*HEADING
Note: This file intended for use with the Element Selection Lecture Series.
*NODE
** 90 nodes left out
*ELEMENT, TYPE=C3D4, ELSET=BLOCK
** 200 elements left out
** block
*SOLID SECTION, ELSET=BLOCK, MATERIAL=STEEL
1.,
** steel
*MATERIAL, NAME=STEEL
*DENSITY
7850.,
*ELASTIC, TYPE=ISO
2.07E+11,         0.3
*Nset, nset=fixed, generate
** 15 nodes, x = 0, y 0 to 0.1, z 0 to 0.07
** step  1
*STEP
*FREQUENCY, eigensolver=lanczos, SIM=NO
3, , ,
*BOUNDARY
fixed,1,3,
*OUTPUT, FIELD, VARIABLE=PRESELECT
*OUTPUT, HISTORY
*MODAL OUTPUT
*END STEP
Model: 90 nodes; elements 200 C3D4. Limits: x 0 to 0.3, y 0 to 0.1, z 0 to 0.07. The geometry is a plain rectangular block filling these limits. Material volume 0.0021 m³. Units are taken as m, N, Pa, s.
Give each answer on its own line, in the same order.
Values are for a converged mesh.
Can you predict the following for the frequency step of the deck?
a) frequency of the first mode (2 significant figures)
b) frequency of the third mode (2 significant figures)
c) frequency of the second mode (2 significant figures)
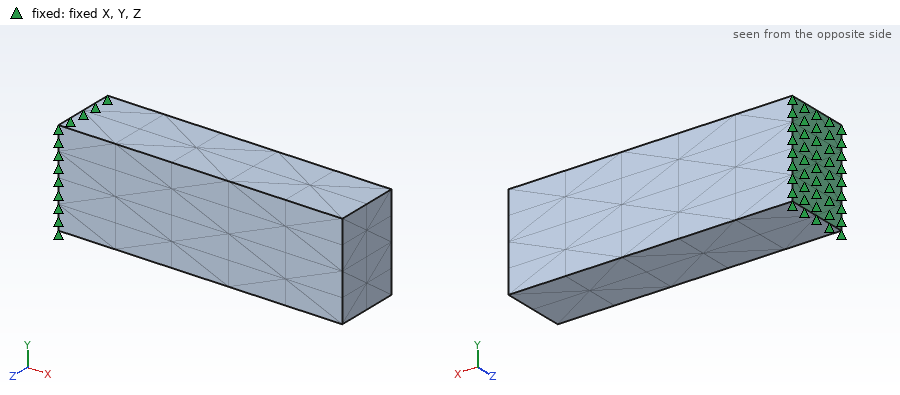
630 Hz
2300 Hz
860 Hz
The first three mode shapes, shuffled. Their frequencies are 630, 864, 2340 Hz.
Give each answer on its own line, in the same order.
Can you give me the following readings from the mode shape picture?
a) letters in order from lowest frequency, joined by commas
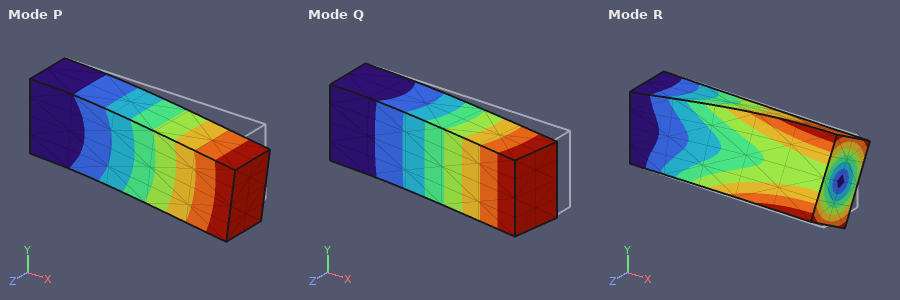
Q, P, R
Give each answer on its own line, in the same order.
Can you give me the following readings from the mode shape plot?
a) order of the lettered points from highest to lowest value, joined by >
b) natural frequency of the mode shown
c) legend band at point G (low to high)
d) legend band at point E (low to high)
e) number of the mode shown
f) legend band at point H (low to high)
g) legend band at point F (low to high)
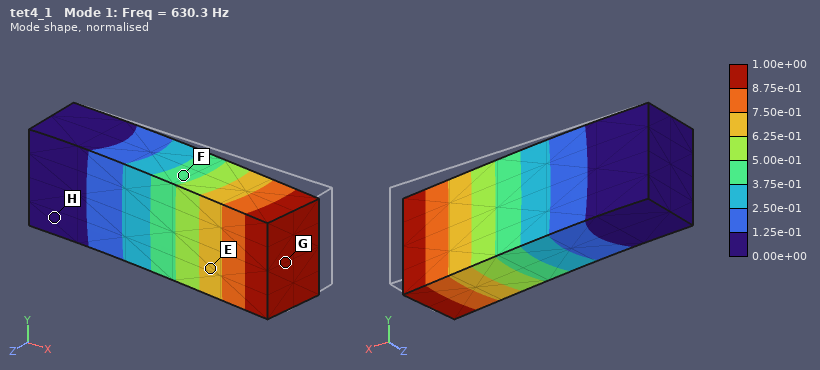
G > E > F > H
630.3 Hz
8.75e-01 to 1.00e+00
6.25e-01 to 7.50e-01
1
0.00e+00 to 1.25e-01
3.75e-01 to 5.00e-01
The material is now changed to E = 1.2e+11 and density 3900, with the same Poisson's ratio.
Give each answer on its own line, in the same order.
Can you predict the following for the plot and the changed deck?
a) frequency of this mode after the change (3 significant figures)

681 Hz
